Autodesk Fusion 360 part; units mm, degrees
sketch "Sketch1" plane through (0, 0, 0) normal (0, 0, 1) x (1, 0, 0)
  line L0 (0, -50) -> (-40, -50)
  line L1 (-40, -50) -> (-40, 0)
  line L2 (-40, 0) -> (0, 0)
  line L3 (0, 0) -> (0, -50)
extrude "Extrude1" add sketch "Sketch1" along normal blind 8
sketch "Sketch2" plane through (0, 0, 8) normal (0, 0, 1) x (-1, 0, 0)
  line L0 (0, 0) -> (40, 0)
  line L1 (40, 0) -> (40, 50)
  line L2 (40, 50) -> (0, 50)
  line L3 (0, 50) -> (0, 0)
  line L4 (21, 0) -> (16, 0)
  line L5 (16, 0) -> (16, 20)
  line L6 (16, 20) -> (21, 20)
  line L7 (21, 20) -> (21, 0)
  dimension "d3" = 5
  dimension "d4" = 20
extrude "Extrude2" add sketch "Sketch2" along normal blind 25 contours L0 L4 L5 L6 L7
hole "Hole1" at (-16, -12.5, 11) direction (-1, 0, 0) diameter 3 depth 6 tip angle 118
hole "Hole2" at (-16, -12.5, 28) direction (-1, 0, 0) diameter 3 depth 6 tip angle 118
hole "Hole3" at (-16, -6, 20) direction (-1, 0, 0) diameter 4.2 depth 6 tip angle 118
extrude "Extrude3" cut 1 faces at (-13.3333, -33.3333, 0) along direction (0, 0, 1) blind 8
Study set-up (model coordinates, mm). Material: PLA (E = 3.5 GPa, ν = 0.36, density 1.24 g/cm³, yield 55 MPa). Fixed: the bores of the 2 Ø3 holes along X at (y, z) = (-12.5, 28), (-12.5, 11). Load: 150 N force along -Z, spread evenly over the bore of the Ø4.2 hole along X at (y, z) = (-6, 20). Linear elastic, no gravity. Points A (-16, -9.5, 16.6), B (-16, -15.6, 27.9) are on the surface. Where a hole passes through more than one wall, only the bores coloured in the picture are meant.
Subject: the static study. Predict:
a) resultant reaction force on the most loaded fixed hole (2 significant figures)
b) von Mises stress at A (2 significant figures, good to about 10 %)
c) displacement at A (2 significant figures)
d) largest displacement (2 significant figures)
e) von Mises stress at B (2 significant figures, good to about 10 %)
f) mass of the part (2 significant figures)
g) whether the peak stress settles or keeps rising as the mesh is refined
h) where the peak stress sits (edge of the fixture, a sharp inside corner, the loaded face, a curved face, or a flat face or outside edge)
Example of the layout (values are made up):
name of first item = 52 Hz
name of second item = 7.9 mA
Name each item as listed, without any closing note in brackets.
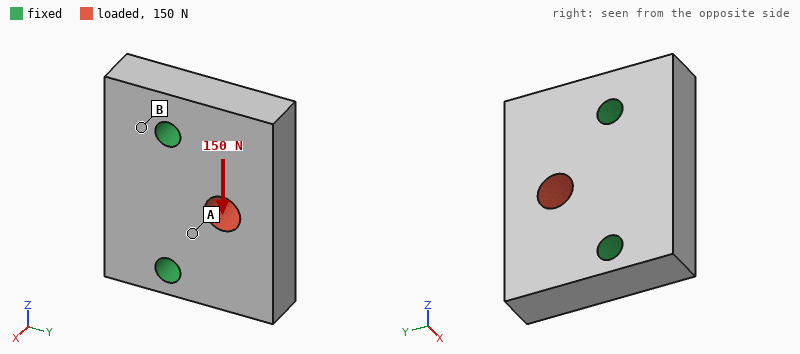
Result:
resultant reaction force on the most loaded fixed hole = 94 N
von Mises stress at A = 2.3 MPa
displacement at A = 3.8 µm
largest displacement = 13 µm
von Mises stress at B = 0.74 MPa
mass of the part = 2.9 g
whether the peak stress settles or keeps rising as the mesh is refined = keeps rising
where the peak stress sits = edge of the fixture
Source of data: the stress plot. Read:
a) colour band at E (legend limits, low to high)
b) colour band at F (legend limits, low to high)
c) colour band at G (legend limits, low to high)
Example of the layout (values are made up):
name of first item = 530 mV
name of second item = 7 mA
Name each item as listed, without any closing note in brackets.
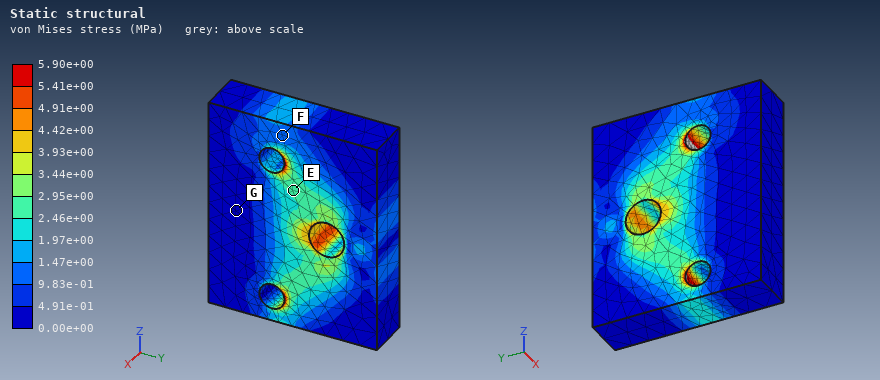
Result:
colour band at E = 2.46e+00 to 2.95e+00 MPa
colour band at F = 9.83e-01 to 1.47e+00 MPa
colour band at G = 0.00e+00 to 4.91e-01 MPa
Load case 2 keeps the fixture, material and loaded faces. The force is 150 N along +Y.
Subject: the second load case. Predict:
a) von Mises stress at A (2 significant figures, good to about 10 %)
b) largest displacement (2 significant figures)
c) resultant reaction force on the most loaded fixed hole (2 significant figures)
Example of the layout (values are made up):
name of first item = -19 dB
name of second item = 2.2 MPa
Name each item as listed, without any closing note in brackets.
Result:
von Mises stress at A = 1.9 MPa
largest displacement = 9.9 µm
resultant reaction force on the most loaded fixed hole = 83 N
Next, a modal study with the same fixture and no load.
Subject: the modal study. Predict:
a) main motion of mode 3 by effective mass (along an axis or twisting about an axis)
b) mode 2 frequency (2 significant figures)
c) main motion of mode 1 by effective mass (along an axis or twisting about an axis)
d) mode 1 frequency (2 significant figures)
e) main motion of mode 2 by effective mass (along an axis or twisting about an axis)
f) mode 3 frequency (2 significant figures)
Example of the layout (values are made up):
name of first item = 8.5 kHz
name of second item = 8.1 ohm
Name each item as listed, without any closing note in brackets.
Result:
main motion of mode 3 by effective mass = along Z
mode 2 frequency = 11 kHz
main motion of mode 1 by effective mass = along X
mode 1 frequency = 7300 Hz
main motion of mode 2 by effective mass = twisting about Y
mode 3 frequency = 15 kHz
